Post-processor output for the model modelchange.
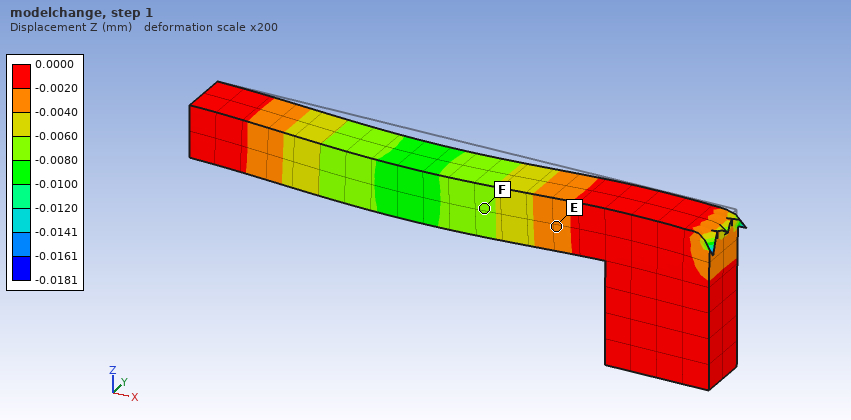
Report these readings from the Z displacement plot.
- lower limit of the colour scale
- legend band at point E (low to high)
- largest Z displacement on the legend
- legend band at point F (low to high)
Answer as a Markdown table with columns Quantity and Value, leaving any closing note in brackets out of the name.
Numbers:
| Quantity | Value |
|---|---|
| lower limit of the colour scale | -0.0181 mm |
| legend band at point E | -0.0040 to -0.0020 mm |
| largest Z displacement on the legend | 0.0000 mm |
| legend band at point F | -0.0080 to -0.0060 mm |
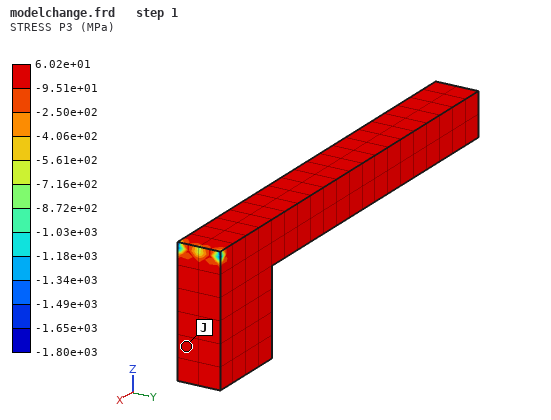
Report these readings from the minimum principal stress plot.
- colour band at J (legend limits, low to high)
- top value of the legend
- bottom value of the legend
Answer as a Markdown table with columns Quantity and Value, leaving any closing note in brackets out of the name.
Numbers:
| Quantity | Value |
|---|---|
| colour band at J | -9.51e+01 to 6.02e+01 MPa |
| top value of the legend | 6.02e+01 MPa |
| bottom value of the legend | -1.80e+03 MPa |
